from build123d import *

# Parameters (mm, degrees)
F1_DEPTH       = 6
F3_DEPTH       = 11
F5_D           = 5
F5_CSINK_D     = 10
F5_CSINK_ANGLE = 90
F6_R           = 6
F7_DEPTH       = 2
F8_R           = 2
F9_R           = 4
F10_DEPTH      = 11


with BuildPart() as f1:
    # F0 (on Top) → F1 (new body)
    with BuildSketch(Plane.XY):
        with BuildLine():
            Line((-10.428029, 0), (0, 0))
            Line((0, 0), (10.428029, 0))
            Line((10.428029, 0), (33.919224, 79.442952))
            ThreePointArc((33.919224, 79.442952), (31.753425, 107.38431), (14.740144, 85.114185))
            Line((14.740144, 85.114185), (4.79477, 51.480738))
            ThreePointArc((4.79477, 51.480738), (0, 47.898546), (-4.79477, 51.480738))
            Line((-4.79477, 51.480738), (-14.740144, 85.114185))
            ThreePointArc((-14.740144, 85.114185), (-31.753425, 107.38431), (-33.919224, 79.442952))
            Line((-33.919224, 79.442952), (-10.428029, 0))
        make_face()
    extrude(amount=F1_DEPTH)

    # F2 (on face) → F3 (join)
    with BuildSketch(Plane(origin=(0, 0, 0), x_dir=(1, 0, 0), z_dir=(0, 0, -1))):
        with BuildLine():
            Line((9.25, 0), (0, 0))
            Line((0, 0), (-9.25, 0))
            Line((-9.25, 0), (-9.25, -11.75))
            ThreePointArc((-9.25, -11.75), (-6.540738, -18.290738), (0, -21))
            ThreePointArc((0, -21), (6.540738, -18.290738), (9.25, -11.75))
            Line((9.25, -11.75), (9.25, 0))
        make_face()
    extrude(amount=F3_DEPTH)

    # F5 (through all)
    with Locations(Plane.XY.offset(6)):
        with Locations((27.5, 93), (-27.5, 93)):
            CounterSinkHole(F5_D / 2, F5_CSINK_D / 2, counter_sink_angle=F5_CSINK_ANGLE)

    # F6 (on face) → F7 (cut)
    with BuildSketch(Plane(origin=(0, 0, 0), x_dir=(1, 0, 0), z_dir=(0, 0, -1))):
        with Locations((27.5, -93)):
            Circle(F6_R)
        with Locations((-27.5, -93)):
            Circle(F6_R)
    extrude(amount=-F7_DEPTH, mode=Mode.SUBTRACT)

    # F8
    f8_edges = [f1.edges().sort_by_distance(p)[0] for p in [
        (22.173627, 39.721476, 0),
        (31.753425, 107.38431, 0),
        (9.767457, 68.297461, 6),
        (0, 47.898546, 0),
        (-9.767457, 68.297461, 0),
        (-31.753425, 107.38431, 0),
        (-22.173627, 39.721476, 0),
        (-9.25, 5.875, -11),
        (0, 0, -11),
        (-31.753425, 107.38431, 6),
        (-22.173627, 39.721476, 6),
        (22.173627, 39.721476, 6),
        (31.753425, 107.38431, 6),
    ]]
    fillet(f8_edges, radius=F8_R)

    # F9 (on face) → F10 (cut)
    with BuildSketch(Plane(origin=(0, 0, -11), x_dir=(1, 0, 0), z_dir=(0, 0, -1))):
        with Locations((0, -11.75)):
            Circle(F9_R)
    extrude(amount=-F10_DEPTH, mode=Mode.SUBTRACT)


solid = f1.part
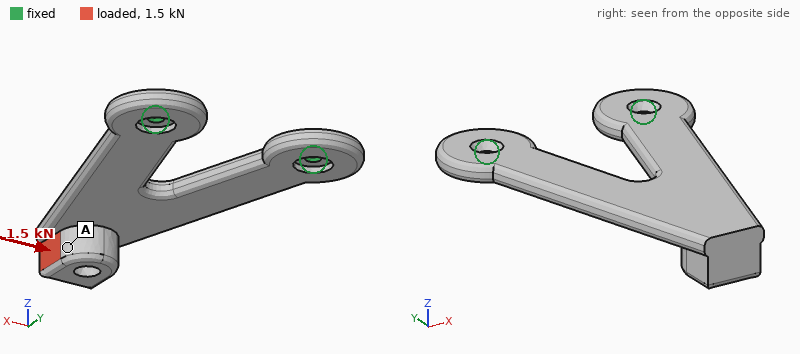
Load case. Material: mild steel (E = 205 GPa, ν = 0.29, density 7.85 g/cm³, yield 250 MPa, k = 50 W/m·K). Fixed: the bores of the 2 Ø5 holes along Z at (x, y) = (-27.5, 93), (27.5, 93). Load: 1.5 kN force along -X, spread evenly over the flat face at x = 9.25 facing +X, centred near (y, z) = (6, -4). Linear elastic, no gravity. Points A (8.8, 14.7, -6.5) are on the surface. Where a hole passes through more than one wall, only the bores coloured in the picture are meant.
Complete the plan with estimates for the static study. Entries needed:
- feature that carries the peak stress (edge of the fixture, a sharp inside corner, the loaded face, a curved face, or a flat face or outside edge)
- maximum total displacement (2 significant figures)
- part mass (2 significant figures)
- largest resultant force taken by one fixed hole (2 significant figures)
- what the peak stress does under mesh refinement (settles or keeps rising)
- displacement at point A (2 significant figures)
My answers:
edge of the fixture
95 µm
220 g
2.4 kN
keeps rising
73 µm
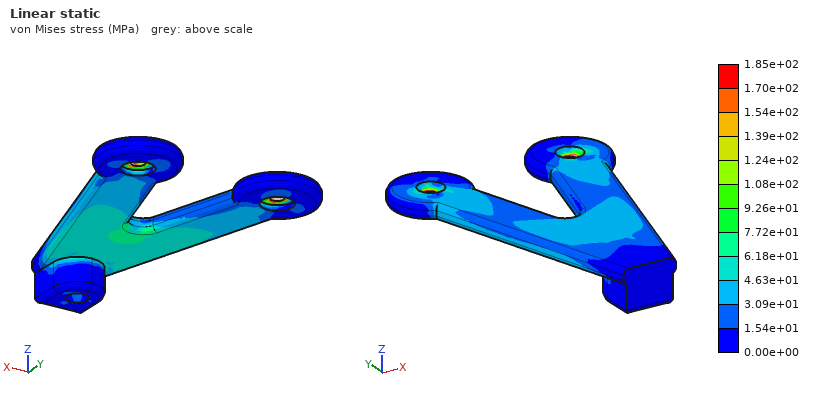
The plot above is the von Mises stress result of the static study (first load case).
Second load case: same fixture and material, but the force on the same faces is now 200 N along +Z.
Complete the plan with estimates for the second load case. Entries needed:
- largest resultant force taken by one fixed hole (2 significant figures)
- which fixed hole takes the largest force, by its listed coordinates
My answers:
120 N
(27.5, 93)
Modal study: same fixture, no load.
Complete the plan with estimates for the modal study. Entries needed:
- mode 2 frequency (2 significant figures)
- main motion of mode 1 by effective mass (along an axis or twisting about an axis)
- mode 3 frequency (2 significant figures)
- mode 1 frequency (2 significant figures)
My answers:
2300 Hz
along Z
2500 Hz
380 Hz
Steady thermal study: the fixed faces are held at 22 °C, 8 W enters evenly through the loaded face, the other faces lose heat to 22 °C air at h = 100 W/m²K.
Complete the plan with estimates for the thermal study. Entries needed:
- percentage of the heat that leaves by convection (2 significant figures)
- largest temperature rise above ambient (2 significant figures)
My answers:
90 %
27 K
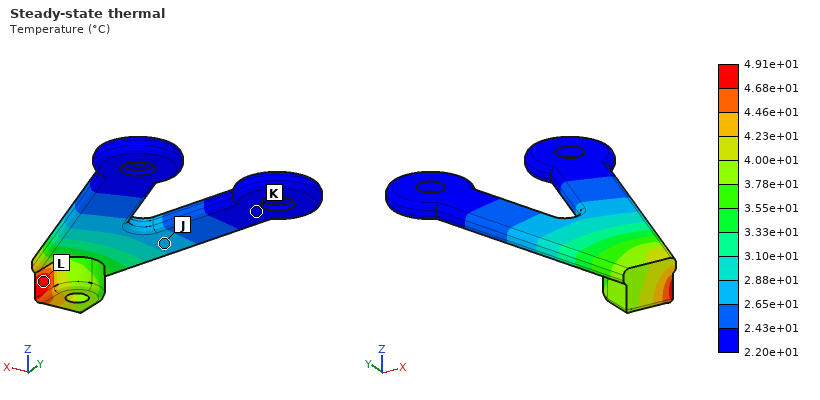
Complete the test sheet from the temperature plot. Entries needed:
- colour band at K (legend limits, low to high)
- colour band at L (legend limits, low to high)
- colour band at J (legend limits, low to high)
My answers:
2.20e+01 to 2.43e+01 °C
4.68e+01 to 4.91e+01 °C
2.65e+01 to 2.88e+01 °C
